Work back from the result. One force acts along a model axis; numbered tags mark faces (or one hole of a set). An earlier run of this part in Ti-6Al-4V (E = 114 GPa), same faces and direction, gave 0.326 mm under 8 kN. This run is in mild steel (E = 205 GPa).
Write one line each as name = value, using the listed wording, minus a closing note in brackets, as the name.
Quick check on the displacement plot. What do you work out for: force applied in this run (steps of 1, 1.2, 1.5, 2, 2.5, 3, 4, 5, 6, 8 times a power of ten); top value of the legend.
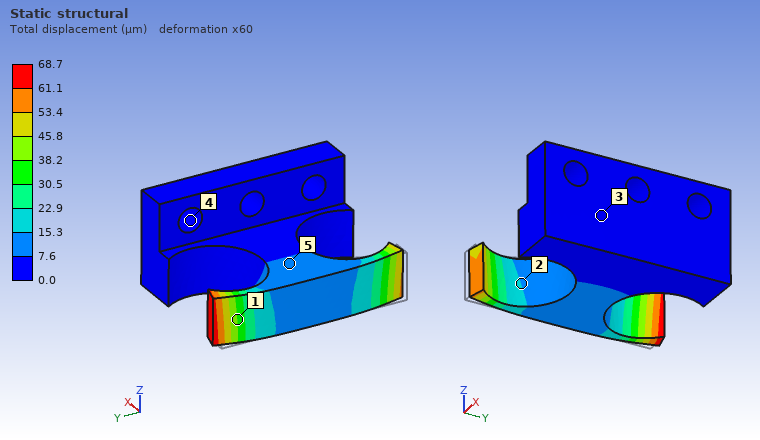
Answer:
force applied in this run = 3 kN
top value of the legend = 68.7 µm
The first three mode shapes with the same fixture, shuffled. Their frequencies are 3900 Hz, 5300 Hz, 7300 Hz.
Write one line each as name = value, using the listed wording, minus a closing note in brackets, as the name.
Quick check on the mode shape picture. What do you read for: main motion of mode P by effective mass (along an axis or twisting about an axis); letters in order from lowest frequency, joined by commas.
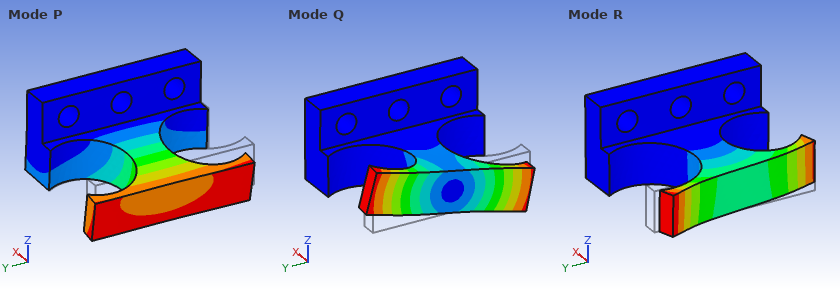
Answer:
main motion of mode P by effective mass = along Z
letters in order from lowest frequency, joined by commas = P, R, Q
